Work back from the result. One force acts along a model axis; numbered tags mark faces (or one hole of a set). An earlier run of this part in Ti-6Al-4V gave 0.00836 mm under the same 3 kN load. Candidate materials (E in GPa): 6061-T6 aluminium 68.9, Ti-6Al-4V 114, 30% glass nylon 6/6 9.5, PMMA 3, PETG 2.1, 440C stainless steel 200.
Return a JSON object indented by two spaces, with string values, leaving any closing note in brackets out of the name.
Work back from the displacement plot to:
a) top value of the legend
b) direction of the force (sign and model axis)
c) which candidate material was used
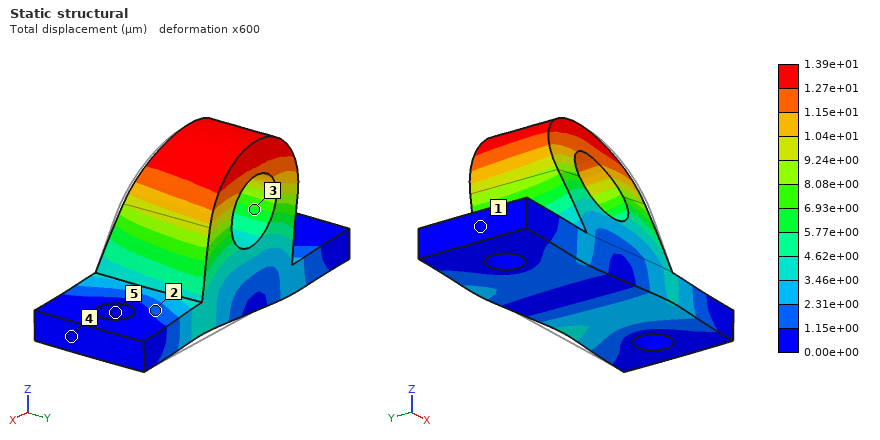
{
  "top value of the legend": "1.39e+01 µm",
  "direction of the force": "-X",
  "which candidate material was used": "6061-T6 aluminium"
}
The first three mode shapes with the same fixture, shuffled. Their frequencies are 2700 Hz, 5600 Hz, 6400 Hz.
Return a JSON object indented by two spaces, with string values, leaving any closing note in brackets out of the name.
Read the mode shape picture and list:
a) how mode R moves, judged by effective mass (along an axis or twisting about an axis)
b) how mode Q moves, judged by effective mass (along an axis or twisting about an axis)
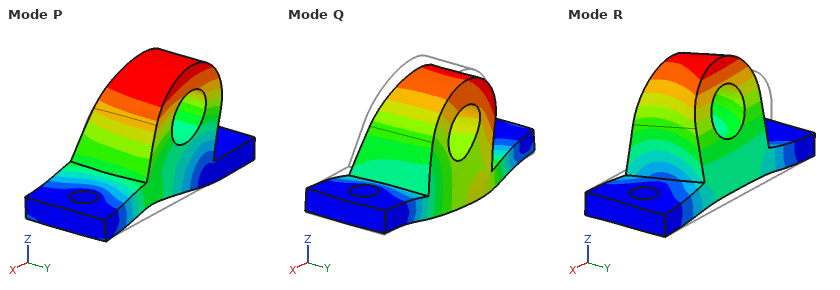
{
  "how mode R moves, judged by effective mass": "along Y",
  "how mode Q moves, judged by effective mass": "along Z"
}
